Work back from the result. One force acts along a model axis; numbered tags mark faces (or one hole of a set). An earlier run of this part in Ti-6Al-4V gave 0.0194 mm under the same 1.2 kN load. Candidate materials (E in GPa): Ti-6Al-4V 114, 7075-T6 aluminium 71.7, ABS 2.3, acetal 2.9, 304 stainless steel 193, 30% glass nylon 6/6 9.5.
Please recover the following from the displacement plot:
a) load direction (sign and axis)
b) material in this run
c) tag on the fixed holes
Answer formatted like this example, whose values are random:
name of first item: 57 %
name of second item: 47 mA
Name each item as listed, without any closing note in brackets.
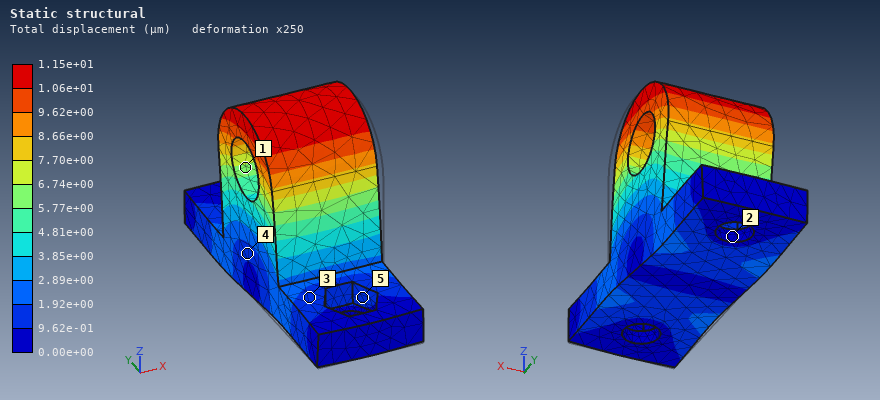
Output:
load direction: +Y
material in this run: 304 stainless steel
tag on the fixed holes: 2
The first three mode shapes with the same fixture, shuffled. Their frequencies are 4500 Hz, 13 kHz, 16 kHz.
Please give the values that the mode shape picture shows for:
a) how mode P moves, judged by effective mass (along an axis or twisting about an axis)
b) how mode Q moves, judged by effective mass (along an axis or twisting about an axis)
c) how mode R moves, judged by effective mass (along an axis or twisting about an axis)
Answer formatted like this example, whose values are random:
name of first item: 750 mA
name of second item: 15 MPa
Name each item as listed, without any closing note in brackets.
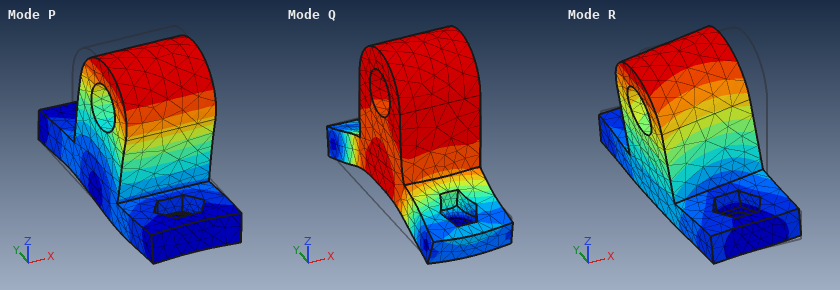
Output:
how mode P moves, judged by effective mass: along Y
how mode Q moves, judged by effective mass: along Z
how mode R moves, judged by effective mass: along X
